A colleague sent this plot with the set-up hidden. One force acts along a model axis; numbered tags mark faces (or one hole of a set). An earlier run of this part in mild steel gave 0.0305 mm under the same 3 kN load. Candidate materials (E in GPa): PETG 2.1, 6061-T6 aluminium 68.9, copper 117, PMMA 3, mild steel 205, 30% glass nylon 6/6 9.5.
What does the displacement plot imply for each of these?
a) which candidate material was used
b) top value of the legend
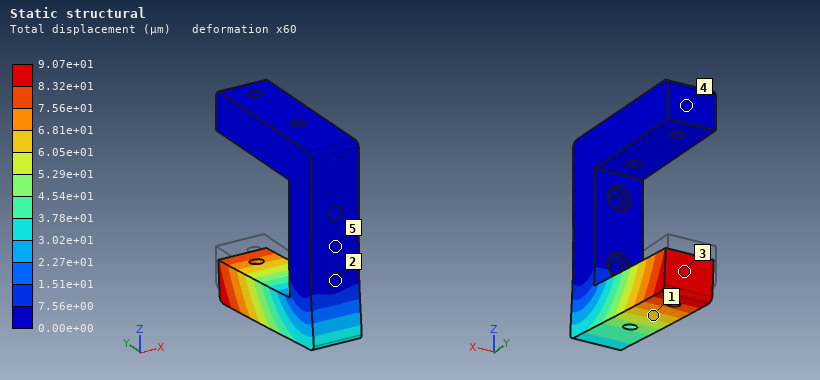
6061-T6 aluminium
9.07e+01 µm
